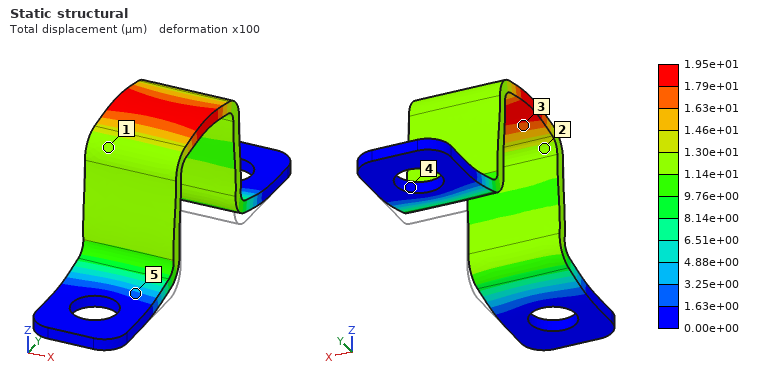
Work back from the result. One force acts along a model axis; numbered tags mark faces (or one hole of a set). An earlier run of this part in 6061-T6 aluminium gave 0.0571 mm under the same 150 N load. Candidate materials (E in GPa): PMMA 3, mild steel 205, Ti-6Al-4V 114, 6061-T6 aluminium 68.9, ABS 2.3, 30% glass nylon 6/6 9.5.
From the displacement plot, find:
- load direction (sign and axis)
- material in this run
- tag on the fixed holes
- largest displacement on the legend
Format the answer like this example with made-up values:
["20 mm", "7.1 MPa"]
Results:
["+Z", "mild steel", "4", "1.95e+01 µm"]
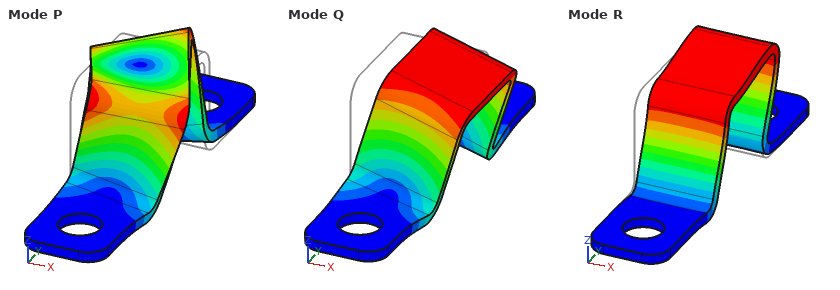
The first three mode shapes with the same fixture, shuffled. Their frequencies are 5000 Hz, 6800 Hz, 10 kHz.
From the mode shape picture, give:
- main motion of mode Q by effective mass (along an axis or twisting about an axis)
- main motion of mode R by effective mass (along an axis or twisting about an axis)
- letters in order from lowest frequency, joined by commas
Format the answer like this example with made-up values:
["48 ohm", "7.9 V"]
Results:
["along X", "along Y", "Q, R, P"]
